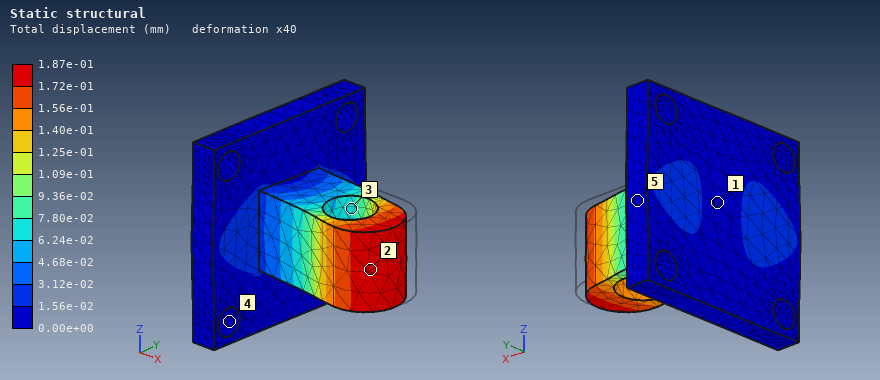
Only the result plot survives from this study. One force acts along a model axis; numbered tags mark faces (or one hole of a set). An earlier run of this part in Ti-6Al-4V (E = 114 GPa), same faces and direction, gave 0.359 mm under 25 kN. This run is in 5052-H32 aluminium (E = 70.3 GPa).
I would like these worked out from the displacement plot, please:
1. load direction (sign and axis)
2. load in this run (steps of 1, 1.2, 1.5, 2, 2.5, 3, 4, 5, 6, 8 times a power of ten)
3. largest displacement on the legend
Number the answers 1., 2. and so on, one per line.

1. -Y
2. 8 kN
3. 1.87e-01 mm
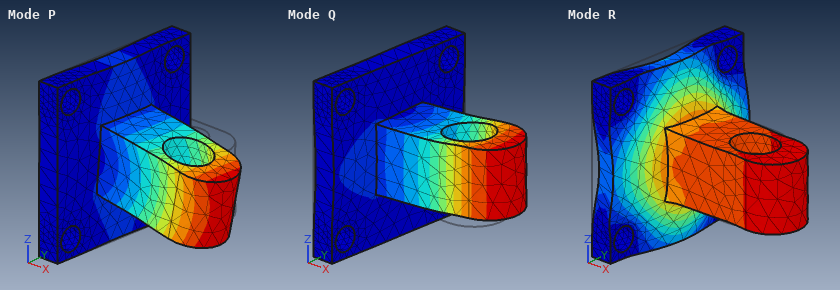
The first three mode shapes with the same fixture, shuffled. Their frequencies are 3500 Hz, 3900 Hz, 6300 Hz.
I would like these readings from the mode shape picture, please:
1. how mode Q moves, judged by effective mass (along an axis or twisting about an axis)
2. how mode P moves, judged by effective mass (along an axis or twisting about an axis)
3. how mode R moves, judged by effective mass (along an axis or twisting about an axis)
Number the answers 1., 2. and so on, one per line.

1. along Y
2. along Z
3. along X
